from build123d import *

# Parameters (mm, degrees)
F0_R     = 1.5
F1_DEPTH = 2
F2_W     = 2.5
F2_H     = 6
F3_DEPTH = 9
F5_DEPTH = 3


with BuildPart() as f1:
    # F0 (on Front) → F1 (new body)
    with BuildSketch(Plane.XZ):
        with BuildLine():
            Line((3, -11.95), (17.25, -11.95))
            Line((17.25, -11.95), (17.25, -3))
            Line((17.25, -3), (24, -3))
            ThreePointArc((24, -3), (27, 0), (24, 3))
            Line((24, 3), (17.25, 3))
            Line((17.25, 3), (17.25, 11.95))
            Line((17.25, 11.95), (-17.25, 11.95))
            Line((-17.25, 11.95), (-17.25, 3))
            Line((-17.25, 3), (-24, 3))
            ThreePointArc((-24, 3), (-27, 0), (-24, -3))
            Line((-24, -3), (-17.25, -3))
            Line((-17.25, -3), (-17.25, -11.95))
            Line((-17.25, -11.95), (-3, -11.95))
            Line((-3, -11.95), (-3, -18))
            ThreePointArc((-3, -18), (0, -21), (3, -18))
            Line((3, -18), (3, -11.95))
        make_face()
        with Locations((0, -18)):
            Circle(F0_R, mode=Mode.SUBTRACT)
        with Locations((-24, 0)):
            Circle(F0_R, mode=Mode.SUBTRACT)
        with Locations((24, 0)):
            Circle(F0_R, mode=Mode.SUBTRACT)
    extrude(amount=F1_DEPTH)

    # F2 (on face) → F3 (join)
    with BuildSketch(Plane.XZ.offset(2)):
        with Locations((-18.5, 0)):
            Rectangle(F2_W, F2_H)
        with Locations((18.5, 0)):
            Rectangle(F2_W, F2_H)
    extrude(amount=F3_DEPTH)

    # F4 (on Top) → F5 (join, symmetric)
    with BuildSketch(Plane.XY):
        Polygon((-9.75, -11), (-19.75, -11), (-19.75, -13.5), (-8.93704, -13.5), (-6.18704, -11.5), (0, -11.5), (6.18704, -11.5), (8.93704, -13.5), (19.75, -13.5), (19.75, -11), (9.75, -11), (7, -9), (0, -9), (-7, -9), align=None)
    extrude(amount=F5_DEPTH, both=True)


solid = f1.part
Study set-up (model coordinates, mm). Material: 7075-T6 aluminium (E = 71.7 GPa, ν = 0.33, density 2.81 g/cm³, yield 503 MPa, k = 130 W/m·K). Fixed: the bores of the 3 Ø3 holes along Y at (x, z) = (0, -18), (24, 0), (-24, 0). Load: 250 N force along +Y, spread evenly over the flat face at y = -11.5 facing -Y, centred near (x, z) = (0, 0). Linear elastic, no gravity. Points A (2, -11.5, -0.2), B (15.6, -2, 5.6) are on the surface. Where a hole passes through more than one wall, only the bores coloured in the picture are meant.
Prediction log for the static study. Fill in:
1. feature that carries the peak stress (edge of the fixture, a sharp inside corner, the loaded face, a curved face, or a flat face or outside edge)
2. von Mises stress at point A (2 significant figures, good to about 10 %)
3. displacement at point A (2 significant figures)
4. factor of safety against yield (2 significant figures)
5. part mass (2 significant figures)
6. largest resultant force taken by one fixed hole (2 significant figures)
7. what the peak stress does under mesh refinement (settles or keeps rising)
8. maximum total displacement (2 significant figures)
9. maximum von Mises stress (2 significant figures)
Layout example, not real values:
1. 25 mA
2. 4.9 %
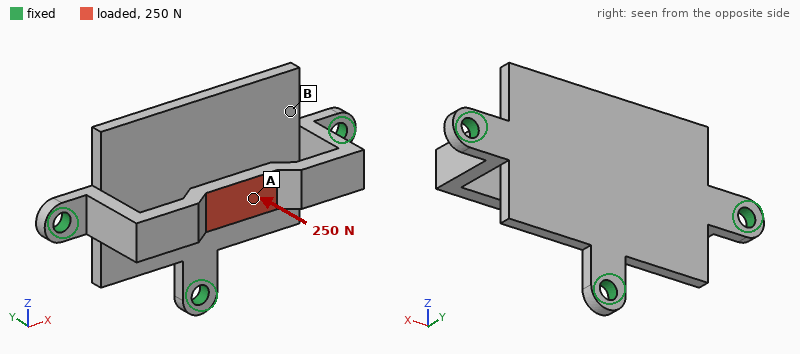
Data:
1. the loaded face
2. 180 MPa
3. 0.19 mm
4. 2.7
5. 7.9 g
6. 150 N
7. settles
8. 0.20 mm
9. 190 MPa
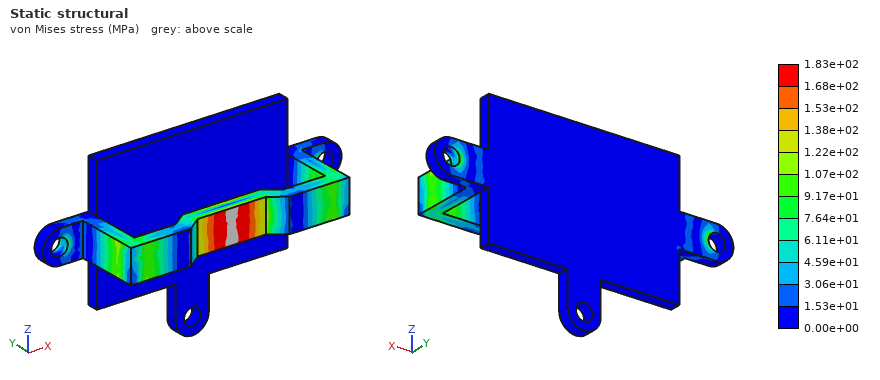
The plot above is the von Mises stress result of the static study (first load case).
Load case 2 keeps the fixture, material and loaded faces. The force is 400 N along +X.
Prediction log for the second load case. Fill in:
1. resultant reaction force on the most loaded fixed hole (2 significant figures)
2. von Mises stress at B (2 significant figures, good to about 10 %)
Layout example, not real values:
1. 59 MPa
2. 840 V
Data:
1. 210 N
2. 34 MPa
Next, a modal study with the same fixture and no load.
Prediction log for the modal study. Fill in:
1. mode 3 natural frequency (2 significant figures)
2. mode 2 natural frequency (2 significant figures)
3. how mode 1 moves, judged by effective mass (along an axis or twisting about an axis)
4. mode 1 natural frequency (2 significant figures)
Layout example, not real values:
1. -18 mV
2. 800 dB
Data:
1. 6000 Hz
2. 5900 Hz
3. along Y
4. 3800 Hz
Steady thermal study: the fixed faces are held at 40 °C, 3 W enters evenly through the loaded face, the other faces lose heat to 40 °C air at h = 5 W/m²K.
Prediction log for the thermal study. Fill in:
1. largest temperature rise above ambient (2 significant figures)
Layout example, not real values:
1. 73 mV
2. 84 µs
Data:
1. 23 K
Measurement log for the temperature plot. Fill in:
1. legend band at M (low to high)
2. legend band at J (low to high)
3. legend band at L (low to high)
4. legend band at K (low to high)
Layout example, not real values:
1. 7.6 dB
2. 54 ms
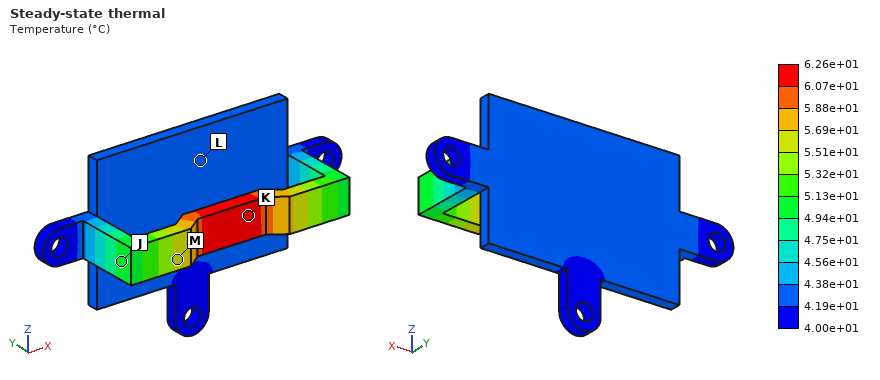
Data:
1. 5.51e+01 to 5.69e+01 °C
2. 4.94e+01 to 5.13e+01 °C
3. 4.19e+01 to 4.38e+01 °C
4. 6.07e+01 to 6.26e+01 °C
